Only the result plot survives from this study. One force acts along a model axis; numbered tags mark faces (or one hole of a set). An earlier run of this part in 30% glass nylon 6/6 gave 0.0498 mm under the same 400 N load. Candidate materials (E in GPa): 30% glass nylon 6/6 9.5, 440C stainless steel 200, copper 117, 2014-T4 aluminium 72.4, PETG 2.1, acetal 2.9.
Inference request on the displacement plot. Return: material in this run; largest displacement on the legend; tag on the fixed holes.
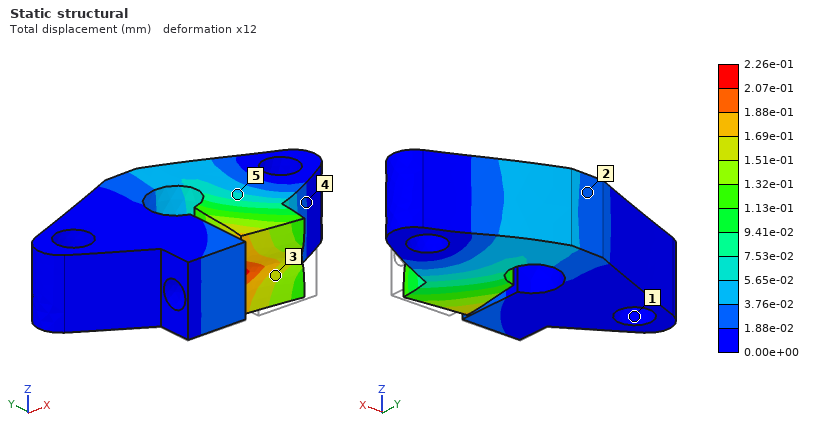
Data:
PETG
2.26e-01 mm
1
